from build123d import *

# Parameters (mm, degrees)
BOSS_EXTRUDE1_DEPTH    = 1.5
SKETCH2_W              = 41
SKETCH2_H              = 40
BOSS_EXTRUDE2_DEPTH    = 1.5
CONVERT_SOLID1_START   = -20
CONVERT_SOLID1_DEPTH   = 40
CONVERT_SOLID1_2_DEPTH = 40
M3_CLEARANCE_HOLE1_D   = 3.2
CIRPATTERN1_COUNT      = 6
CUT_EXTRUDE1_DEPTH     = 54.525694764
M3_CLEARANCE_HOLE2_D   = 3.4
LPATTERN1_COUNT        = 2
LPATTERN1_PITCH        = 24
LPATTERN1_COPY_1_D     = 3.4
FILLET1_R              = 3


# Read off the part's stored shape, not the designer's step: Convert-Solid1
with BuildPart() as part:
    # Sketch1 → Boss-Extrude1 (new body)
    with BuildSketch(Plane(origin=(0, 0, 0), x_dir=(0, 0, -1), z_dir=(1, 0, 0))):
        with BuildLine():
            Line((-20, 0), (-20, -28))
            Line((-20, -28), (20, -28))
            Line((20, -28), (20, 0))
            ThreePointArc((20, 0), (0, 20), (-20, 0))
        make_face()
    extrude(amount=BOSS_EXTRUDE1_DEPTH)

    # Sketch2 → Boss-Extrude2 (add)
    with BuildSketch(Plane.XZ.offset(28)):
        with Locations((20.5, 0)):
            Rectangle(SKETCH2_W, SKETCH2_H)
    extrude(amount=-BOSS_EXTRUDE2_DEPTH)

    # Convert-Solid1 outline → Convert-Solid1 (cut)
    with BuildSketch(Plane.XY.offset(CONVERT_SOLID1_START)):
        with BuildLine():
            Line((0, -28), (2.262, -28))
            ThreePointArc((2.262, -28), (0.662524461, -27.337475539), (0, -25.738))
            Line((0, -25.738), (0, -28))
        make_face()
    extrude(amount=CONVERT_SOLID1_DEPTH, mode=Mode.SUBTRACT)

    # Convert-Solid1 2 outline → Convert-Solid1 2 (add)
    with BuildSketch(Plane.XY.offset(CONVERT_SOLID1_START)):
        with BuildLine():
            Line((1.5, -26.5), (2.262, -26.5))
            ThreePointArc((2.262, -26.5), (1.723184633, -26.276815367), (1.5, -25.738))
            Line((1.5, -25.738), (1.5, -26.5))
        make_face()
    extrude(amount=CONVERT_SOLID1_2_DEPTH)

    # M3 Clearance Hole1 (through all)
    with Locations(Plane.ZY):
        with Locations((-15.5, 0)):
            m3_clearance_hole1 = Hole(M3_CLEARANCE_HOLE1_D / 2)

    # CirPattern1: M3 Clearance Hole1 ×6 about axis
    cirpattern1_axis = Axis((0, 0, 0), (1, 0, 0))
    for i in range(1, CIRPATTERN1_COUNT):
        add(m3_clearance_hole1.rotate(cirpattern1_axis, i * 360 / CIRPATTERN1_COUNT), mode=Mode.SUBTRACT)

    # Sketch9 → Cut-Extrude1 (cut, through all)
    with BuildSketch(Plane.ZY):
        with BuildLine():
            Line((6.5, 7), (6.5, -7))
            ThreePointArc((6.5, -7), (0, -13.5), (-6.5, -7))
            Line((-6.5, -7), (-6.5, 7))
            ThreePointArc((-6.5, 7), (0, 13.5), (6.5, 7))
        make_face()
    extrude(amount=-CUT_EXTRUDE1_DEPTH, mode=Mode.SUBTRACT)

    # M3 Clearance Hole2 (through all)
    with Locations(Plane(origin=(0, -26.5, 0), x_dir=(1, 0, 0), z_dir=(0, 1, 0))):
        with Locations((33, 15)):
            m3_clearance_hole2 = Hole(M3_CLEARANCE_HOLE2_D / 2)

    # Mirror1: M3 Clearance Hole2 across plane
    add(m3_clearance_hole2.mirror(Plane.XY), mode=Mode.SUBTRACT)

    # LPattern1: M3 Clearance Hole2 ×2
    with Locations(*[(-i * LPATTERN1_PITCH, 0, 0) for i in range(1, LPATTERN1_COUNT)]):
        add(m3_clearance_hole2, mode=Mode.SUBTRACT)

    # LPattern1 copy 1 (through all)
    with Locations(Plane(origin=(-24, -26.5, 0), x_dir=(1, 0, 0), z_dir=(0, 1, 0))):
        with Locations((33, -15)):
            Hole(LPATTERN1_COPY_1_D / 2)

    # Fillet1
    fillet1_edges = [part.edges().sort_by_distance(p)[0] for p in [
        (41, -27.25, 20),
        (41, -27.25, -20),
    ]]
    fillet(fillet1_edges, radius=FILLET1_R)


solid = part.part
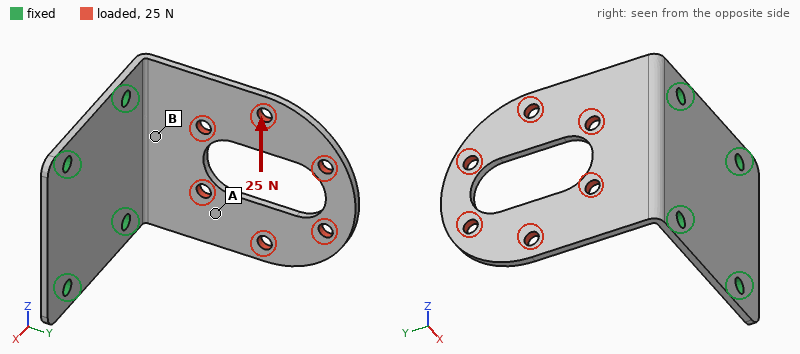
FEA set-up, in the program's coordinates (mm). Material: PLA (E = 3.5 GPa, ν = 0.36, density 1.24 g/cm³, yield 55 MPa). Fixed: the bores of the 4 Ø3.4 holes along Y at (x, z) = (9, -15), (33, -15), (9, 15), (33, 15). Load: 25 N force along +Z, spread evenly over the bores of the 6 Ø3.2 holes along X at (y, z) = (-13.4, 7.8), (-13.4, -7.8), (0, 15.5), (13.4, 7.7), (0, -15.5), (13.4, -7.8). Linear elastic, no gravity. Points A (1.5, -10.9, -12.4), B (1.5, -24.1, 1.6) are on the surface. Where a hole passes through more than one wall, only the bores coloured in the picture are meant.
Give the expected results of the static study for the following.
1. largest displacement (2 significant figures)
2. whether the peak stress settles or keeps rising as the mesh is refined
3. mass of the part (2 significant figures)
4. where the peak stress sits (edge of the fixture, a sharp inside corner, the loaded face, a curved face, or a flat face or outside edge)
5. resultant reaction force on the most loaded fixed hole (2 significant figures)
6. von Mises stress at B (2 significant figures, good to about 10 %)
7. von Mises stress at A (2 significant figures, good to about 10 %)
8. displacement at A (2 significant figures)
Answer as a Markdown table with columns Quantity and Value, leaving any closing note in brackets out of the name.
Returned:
| Quantity | Value |
|---|---|
| largest displacement | 0.59 mm |
| whether the peak stress settles or keeps rising as the mesh is refined | keeps rising |
| mass of the part | 5.4 g |
| where the peak stress sits | edge of the fixture |
| resultant reaction force on the most loaded fixed hole | 26 N |
| von Mises stress at B | 5.6 MPa |
| von Mises stress at A | 2.1 MPa |
| displacement at A | 0.30 mm |
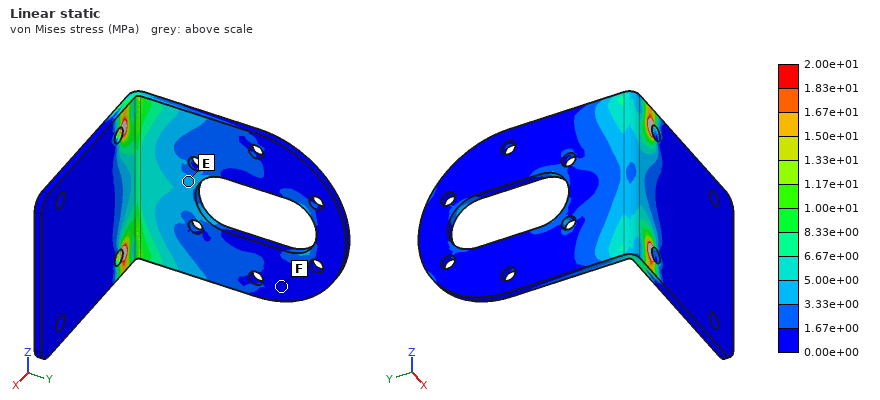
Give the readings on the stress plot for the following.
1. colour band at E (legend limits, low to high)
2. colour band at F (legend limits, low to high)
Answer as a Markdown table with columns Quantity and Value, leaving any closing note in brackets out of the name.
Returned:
| Quantity | Value |
|---|---|
| colour band at E | 3.33e+00 to 5.00e+00 MPa |
| colour band at F | 0.00e+00 to 1.67e+00 MPa |
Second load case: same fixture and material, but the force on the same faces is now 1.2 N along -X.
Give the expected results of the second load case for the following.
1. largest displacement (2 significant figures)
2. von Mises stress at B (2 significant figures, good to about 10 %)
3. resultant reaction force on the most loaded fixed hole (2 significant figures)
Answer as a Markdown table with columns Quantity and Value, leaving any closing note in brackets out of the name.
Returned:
| Quantity | Value |
|---|---|
| largest displacement | 0.80 mm |
| von Mises stress at B | 1.7 MPa |
| resultant reaction force on the most loaded fixed hole | 0.40 N |
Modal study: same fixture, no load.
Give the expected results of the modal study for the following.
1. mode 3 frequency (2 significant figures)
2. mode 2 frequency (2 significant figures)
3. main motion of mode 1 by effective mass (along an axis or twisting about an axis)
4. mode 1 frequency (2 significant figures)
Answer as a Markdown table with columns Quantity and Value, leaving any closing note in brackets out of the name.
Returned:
| Quantity | Value |
|---|---|
| mode 3 frequency | 950 Hz |
| mode 2 frequency | 510 Hz |
| main motion of mode 1 by effective mass | along X |
| mode 1 frequency | 190 Hz |
